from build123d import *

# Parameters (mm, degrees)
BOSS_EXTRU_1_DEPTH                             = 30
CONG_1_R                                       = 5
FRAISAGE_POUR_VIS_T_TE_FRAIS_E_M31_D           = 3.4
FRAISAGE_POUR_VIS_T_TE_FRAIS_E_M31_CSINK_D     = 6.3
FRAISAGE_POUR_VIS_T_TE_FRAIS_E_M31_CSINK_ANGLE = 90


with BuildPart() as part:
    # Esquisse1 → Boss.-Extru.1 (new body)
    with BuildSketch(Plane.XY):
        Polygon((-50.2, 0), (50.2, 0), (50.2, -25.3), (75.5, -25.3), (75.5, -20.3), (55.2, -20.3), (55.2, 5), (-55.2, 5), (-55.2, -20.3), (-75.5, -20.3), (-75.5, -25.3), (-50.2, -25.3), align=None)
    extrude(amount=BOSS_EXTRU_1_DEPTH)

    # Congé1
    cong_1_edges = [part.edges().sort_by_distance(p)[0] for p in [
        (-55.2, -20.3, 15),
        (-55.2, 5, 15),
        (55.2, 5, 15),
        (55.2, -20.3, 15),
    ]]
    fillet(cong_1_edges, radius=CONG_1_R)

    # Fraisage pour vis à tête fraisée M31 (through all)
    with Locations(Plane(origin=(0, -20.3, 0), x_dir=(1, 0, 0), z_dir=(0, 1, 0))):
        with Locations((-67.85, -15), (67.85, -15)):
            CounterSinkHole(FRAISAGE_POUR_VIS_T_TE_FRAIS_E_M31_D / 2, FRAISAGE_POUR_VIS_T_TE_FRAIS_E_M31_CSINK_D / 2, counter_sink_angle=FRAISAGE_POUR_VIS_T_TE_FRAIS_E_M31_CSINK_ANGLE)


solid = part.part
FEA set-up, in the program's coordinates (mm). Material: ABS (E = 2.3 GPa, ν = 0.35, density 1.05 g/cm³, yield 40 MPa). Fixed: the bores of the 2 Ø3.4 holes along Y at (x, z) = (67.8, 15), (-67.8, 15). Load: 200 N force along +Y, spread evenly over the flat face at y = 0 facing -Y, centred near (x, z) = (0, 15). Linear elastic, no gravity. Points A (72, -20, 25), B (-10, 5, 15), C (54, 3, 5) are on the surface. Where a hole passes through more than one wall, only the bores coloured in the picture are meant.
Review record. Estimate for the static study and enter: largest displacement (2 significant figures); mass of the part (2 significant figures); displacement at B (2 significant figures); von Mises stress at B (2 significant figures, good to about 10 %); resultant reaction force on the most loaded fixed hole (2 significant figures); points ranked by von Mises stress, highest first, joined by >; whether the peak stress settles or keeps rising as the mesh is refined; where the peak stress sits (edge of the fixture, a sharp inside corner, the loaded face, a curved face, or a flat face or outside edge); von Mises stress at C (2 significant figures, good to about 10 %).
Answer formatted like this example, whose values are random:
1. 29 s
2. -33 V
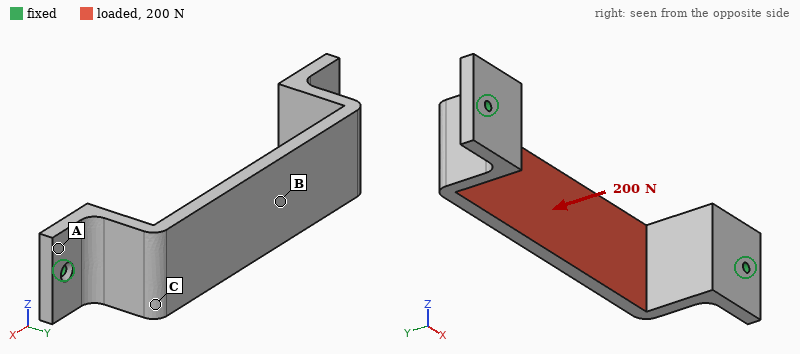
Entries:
1. 1.2 mm
2. 32 g
3. 1.1 mm
4. 8.1 MPa
5. 150 N
6. B > C > A
7. keeps rising
8. edge of the fixture
9. 5.1 MPa
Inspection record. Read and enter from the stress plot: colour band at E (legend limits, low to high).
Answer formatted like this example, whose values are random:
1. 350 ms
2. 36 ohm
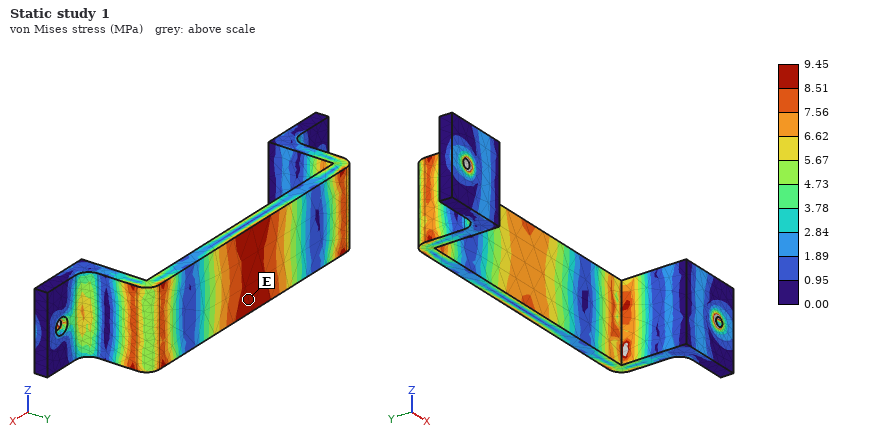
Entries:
1. 8.51 to 9.45 MPa
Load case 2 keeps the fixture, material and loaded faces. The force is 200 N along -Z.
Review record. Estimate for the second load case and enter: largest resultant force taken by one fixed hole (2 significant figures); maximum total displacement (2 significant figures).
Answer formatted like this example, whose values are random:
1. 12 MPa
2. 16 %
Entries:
1. 100 N
2. 1.6 mm
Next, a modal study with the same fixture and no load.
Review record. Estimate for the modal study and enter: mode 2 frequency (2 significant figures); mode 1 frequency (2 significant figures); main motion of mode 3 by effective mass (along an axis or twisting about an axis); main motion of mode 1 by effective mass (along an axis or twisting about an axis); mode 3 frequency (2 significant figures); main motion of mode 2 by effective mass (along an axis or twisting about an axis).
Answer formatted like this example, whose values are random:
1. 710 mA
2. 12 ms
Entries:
1. 520 Hz
2. 390 Hz
3. along Y
4. along Z
5. 590 Hz
6. along X
